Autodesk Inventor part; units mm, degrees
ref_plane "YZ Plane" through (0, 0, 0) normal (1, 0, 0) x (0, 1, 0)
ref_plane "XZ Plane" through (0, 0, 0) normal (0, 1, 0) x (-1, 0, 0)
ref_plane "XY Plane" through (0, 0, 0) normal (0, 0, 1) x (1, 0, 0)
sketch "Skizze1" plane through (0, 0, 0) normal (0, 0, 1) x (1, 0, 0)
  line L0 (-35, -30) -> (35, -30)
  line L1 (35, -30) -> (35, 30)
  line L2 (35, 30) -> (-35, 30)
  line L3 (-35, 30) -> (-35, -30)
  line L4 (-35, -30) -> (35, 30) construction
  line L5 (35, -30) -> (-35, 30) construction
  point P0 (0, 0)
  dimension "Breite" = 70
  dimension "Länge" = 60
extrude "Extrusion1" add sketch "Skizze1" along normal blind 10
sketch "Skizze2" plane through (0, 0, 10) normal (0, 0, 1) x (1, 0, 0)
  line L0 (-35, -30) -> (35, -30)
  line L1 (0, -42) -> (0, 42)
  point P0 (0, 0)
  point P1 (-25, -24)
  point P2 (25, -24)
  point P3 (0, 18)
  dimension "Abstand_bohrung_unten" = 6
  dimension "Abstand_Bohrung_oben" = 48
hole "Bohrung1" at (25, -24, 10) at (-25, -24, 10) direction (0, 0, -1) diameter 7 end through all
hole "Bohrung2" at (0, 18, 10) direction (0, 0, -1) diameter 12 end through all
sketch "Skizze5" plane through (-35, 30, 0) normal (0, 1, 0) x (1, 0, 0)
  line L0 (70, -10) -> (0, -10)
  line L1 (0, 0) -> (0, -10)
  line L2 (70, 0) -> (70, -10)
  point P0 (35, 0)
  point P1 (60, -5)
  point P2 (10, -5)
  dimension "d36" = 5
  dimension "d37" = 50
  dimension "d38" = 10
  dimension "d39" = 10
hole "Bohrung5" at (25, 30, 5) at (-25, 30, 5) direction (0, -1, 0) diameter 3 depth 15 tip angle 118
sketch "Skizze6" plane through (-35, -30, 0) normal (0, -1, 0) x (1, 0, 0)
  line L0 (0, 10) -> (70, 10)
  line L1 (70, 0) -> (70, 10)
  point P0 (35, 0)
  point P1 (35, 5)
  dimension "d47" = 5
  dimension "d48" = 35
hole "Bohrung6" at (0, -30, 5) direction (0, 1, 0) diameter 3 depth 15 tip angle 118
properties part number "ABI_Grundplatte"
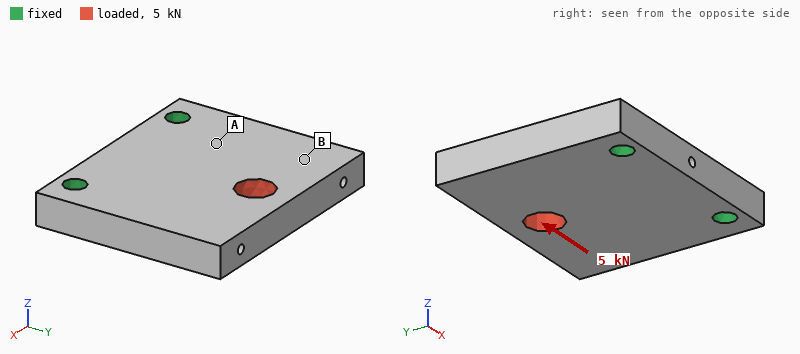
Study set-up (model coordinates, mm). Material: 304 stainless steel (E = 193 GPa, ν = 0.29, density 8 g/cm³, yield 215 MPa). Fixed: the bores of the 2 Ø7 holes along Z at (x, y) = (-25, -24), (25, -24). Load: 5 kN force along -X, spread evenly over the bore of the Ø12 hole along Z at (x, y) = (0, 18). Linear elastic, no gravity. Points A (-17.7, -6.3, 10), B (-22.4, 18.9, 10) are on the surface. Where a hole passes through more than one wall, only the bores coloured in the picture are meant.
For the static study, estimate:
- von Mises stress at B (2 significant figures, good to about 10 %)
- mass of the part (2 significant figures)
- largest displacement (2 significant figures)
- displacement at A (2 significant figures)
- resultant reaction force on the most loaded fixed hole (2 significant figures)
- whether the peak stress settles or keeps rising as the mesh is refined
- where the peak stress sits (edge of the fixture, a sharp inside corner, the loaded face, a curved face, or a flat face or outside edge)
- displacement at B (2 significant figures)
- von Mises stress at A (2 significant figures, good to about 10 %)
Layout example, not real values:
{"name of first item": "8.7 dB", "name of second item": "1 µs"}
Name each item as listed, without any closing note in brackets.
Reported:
{"von Mises stress at B": "6.7 MPa", "mass of the part": "320 g", "largest displacement": "10 µm", "displacement at A": "2.9 µm", "resultant reaction force on the most loaded fixed hole": "4.6 kN", "whether the peak stress settles or keeps rising as the mesh is refined": "keeps rising", "where the peak stress sits": "edge of the fixture", "displacement at B": "7.8 µm", "von Mises stress at A": "17 MPa"}
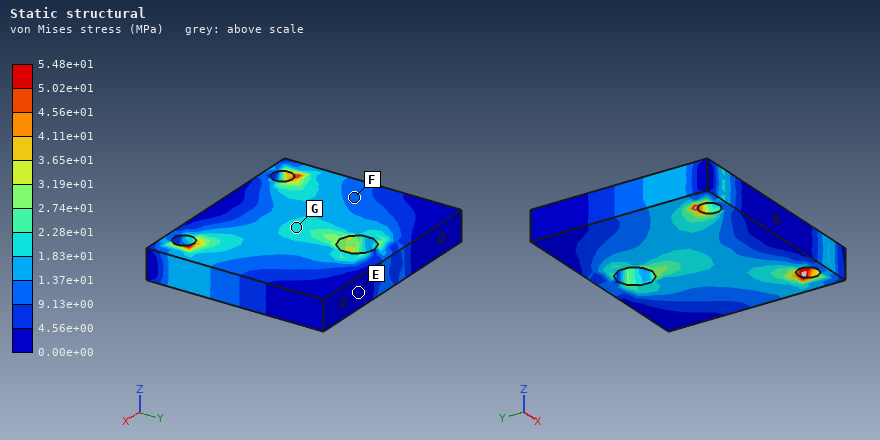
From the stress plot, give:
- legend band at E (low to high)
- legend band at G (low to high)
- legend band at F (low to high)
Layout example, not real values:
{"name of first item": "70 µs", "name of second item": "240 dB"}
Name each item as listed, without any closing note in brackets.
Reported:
{"legend band at E": "0.00e+00 to 4.56e+00 MPa", "legend band at G": "1.83e+01 to 2.28e+01 MPa", "legend band at F": "9.13e+00 to 1.37e+01 MPa"}
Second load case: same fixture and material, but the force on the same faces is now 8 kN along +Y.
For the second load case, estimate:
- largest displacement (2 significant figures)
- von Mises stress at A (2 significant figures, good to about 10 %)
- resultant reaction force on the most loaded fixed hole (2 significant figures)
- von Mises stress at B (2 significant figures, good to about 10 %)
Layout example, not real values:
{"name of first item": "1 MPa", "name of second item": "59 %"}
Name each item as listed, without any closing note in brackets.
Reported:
{"largest displacement": "7.5 µm", "von Mises stress at A": "19 MPa", "resultant reaction force on the most loaded fixed hole": "4.2 kN", "von Mises stress at B": "4.7 MPa"}
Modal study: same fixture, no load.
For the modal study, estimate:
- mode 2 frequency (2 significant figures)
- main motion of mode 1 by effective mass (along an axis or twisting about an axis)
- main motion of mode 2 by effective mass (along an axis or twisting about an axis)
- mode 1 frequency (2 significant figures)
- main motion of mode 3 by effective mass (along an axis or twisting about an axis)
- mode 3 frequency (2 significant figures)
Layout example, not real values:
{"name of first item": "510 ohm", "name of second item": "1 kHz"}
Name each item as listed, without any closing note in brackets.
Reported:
{"mode 2 frequency": "5100 Hz", "main motion of mode 1 by effective mass": "along Z", "main motion of mode 2 by effective mass": "twisting about Y", "mode 1 frequency": "2500 Hz", "main motion of mode 3 by effective mass": "along X", "mode 3 frequency": "10 kHz"}
